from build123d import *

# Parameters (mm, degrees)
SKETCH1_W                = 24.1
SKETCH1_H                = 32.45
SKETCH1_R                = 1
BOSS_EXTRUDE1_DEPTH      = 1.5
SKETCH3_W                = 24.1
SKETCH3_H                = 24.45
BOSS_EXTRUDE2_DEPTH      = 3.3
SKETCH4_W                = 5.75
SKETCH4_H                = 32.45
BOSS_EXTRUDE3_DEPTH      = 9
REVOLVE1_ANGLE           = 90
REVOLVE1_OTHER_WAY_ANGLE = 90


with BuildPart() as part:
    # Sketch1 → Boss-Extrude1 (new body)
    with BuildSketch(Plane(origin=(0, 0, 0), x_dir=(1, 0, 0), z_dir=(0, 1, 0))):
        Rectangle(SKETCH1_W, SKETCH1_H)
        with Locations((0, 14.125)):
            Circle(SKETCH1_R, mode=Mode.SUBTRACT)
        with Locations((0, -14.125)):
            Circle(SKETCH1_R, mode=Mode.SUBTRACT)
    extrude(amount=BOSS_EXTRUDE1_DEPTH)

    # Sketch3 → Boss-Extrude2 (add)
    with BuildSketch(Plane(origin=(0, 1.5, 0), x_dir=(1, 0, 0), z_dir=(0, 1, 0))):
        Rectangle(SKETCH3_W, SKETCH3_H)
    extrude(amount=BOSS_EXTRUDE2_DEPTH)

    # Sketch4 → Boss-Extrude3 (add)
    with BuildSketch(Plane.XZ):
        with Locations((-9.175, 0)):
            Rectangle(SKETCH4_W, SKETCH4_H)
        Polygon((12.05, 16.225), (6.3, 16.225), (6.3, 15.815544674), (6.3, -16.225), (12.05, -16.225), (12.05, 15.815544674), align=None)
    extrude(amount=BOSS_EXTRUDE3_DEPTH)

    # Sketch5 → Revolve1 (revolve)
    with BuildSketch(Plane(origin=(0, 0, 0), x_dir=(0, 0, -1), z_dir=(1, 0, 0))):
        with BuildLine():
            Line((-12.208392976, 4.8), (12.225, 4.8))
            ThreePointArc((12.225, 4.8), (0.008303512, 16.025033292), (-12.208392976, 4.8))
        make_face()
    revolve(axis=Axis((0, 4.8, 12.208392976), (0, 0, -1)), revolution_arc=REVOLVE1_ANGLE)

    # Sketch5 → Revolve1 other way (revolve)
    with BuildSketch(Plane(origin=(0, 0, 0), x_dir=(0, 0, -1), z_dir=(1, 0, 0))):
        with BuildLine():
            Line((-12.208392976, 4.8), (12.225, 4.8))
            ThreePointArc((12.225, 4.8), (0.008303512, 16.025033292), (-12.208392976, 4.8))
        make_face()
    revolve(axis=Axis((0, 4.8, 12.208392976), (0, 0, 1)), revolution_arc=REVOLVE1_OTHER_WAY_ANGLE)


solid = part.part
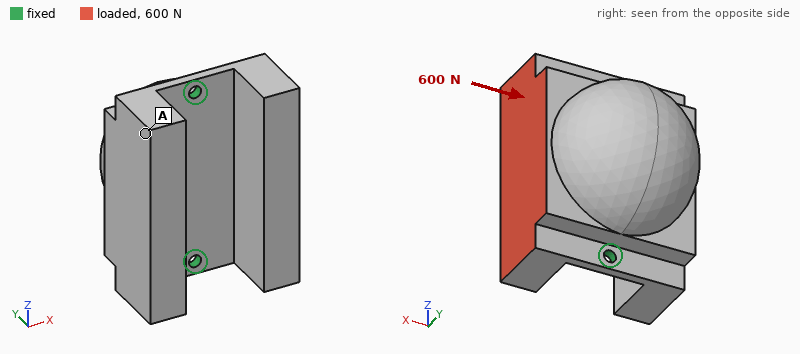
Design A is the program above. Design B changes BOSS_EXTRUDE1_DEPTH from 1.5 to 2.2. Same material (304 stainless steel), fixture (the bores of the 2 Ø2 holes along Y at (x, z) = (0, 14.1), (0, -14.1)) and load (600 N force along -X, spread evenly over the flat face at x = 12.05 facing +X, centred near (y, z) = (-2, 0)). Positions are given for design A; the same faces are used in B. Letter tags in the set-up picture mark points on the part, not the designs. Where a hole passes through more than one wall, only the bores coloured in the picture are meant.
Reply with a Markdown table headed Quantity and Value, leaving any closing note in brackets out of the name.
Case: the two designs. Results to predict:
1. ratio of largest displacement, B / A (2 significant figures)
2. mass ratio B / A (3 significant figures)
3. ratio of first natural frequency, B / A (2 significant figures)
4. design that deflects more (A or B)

| Quantity | Value |
|---|---|
| ratio of largest displacement, B / A | 0.55 |
| mass ratio B / A | 1.01 |
| ratio of first natural frequency, B / A | 1.5 |
| design that deflects more | A |
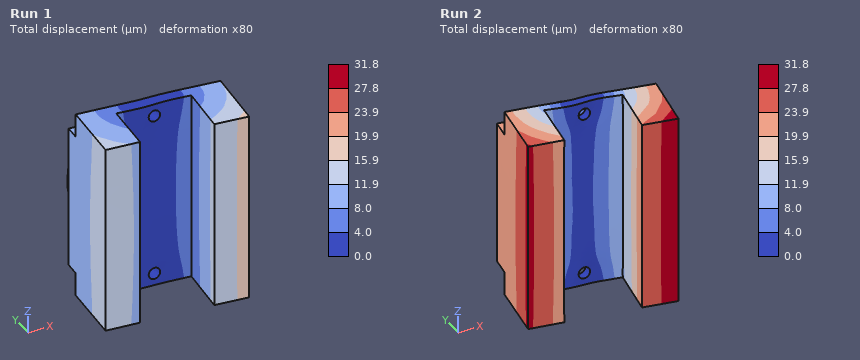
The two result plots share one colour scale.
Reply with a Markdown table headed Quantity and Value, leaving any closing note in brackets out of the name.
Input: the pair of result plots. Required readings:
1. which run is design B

| Quantity | Value |
|---|---|
| which run is design B | Run 1 |
